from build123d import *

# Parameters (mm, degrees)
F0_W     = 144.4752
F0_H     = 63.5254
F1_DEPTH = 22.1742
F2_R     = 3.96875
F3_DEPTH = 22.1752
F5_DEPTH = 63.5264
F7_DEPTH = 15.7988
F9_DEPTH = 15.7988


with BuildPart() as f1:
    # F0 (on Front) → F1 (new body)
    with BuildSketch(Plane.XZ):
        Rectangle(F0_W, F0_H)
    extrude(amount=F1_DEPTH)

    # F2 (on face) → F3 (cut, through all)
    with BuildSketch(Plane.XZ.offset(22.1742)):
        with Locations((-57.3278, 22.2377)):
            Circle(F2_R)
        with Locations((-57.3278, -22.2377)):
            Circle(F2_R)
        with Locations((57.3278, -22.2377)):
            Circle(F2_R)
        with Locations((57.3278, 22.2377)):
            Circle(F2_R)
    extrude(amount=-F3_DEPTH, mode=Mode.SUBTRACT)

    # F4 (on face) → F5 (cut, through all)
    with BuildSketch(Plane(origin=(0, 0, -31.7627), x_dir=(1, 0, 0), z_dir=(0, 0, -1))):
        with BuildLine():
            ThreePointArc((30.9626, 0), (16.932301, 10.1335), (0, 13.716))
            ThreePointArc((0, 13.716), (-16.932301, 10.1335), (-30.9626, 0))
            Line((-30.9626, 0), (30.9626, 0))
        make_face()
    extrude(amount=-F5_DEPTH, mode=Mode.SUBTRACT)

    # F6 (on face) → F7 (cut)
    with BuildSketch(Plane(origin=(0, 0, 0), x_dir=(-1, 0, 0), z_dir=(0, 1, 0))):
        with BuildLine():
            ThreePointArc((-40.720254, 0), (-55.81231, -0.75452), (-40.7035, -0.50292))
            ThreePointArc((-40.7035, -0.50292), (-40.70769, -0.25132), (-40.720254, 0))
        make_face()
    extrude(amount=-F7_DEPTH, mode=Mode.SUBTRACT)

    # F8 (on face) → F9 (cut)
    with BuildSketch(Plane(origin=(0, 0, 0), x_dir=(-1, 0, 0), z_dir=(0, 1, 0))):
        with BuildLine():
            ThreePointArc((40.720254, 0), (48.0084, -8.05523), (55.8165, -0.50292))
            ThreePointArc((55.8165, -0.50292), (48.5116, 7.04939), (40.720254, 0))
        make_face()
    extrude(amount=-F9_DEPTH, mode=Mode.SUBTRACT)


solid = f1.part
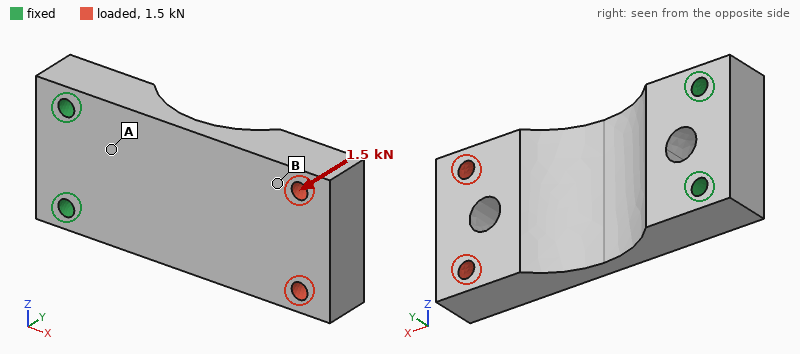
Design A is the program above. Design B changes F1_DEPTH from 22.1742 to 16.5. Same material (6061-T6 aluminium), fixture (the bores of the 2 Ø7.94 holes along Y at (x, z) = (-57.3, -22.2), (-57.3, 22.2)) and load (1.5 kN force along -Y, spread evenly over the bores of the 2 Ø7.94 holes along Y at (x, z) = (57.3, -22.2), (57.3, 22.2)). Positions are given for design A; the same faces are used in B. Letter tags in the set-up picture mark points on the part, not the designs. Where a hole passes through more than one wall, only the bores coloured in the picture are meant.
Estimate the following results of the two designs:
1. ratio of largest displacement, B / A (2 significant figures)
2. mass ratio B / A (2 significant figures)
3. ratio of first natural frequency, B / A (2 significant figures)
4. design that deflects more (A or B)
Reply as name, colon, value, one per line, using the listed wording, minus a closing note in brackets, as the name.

ratio of largest displacement, B / A: 13
mass ratio B / A: 0.67
ratio of first natural frequency, B / A: 0.33
design that deflects more: B
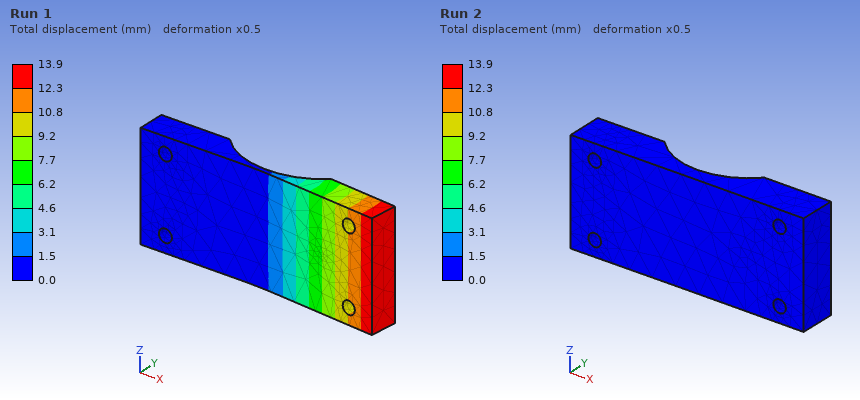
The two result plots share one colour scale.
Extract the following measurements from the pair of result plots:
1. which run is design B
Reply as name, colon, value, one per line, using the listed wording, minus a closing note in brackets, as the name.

which run is design B: Run 1
